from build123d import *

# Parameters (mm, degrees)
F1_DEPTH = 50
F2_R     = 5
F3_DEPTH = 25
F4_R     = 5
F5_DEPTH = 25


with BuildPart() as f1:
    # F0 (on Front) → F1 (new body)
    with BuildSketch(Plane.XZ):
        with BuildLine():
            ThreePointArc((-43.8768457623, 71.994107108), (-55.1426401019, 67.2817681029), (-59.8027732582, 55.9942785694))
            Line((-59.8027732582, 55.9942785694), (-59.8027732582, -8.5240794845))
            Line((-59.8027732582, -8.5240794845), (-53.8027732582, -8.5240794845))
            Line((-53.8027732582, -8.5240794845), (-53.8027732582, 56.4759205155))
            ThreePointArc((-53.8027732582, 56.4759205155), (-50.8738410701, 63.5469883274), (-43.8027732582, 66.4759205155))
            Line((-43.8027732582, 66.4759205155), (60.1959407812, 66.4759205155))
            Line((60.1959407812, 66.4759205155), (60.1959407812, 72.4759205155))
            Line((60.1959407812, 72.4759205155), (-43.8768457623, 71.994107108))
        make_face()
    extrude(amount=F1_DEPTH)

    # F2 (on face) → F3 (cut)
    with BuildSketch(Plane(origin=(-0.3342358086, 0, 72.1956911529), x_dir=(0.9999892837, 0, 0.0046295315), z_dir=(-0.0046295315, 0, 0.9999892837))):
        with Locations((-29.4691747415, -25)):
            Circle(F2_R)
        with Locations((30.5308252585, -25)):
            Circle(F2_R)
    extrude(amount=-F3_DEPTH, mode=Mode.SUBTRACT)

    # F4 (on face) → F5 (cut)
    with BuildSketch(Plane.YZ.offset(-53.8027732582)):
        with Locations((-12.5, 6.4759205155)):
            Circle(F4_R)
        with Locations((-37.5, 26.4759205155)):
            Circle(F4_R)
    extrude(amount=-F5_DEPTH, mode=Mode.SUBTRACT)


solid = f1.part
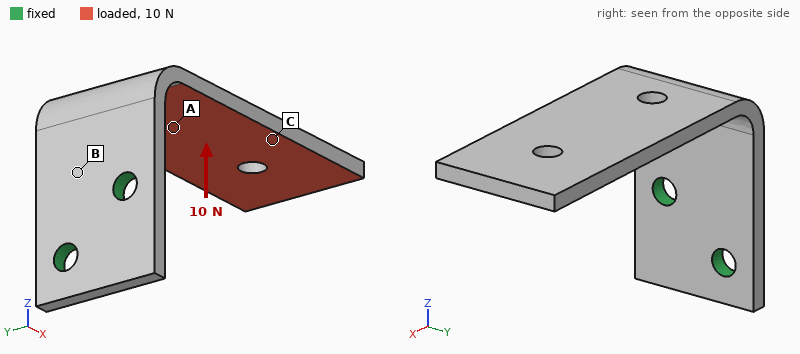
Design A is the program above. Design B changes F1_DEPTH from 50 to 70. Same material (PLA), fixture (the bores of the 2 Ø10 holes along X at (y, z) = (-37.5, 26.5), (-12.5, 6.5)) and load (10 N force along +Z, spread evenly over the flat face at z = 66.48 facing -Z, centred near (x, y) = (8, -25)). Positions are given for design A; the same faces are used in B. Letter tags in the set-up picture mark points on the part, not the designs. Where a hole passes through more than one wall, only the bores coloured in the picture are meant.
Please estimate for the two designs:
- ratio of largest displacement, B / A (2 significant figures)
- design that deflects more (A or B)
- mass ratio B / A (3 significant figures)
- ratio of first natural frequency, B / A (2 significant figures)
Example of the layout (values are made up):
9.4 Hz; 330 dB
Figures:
0.71; A; 1.41; 1.0
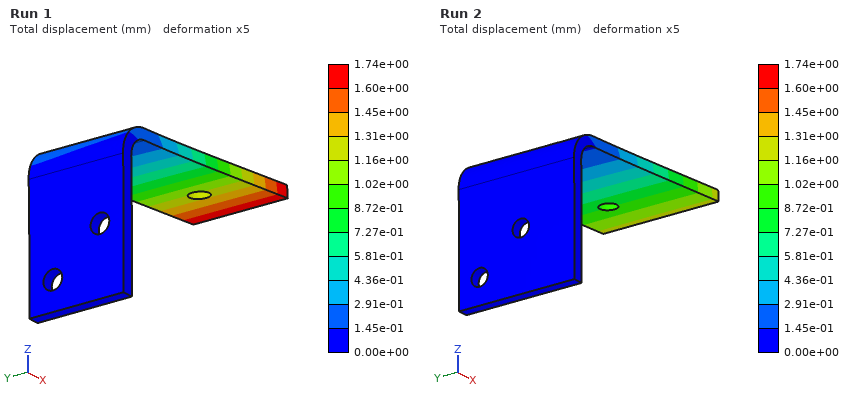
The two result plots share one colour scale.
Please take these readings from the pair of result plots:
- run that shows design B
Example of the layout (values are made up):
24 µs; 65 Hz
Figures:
Run 2
